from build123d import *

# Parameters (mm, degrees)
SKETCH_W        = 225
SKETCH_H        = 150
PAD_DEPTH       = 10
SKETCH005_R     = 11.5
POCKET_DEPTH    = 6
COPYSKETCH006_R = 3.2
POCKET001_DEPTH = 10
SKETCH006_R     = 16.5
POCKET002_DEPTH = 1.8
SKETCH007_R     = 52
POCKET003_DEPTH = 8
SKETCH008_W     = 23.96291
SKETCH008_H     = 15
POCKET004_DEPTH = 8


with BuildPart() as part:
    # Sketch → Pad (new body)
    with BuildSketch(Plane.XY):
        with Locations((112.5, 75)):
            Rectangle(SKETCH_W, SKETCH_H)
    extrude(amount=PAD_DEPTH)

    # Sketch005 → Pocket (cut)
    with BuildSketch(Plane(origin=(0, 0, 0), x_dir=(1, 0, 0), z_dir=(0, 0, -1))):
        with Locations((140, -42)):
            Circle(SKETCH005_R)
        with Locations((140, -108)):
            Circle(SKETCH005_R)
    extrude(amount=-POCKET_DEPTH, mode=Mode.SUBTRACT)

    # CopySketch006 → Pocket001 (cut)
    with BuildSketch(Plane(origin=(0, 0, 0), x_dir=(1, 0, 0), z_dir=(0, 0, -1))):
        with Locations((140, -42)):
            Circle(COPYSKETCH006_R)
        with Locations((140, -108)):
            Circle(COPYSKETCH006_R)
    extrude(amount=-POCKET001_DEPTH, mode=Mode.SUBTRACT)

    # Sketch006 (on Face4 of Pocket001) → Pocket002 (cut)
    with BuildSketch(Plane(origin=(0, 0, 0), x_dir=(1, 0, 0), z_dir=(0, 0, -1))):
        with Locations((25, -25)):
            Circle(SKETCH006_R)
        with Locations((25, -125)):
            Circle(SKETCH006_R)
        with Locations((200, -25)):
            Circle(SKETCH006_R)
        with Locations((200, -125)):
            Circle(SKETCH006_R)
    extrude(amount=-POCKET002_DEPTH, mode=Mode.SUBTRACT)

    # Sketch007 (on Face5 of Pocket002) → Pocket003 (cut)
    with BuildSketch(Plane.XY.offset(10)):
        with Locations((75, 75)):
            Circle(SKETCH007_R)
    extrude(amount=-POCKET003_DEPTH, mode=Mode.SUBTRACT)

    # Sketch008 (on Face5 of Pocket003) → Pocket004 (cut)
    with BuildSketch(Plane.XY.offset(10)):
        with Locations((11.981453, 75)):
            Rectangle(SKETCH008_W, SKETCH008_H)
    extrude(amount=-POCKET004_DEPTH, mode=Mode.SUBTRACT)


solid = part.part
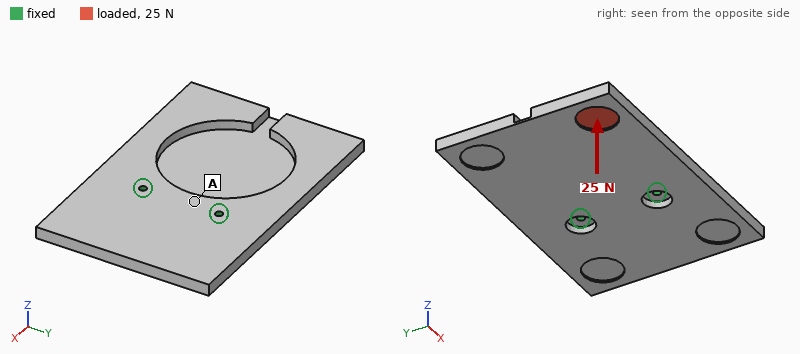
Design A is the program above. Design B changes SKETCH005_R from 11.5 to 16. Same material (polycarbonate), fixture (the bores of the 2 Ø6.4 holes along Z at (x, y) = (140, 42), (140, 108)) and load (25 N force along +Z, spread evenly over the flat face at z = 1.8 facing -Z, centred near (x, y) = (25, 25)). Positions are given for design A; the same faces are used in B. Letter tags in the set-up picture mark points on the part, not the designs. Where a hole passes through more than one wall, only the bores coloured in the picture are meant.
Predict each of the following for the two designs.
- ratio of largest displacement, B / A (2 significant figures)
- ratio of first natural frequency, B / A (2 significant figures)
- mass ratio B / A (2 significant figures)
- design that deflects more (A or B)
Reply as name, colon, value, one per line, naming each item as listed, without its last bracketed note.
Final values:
ratio of largest displacement, B / A: 1.1
ratio of first natural frequency, B / A: 0.93
mass ratio B / A: 0.98
design that deflects more: B
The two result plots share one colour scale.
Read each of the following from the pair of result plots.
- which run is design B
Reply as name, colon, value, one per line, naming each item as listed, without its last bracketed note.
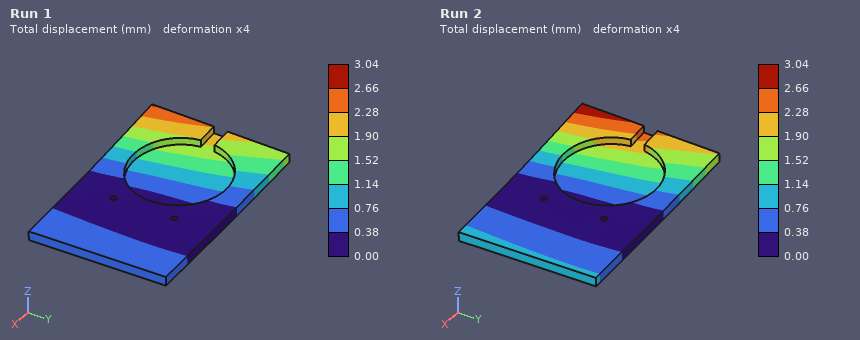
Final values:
which run is design B: Run 2
